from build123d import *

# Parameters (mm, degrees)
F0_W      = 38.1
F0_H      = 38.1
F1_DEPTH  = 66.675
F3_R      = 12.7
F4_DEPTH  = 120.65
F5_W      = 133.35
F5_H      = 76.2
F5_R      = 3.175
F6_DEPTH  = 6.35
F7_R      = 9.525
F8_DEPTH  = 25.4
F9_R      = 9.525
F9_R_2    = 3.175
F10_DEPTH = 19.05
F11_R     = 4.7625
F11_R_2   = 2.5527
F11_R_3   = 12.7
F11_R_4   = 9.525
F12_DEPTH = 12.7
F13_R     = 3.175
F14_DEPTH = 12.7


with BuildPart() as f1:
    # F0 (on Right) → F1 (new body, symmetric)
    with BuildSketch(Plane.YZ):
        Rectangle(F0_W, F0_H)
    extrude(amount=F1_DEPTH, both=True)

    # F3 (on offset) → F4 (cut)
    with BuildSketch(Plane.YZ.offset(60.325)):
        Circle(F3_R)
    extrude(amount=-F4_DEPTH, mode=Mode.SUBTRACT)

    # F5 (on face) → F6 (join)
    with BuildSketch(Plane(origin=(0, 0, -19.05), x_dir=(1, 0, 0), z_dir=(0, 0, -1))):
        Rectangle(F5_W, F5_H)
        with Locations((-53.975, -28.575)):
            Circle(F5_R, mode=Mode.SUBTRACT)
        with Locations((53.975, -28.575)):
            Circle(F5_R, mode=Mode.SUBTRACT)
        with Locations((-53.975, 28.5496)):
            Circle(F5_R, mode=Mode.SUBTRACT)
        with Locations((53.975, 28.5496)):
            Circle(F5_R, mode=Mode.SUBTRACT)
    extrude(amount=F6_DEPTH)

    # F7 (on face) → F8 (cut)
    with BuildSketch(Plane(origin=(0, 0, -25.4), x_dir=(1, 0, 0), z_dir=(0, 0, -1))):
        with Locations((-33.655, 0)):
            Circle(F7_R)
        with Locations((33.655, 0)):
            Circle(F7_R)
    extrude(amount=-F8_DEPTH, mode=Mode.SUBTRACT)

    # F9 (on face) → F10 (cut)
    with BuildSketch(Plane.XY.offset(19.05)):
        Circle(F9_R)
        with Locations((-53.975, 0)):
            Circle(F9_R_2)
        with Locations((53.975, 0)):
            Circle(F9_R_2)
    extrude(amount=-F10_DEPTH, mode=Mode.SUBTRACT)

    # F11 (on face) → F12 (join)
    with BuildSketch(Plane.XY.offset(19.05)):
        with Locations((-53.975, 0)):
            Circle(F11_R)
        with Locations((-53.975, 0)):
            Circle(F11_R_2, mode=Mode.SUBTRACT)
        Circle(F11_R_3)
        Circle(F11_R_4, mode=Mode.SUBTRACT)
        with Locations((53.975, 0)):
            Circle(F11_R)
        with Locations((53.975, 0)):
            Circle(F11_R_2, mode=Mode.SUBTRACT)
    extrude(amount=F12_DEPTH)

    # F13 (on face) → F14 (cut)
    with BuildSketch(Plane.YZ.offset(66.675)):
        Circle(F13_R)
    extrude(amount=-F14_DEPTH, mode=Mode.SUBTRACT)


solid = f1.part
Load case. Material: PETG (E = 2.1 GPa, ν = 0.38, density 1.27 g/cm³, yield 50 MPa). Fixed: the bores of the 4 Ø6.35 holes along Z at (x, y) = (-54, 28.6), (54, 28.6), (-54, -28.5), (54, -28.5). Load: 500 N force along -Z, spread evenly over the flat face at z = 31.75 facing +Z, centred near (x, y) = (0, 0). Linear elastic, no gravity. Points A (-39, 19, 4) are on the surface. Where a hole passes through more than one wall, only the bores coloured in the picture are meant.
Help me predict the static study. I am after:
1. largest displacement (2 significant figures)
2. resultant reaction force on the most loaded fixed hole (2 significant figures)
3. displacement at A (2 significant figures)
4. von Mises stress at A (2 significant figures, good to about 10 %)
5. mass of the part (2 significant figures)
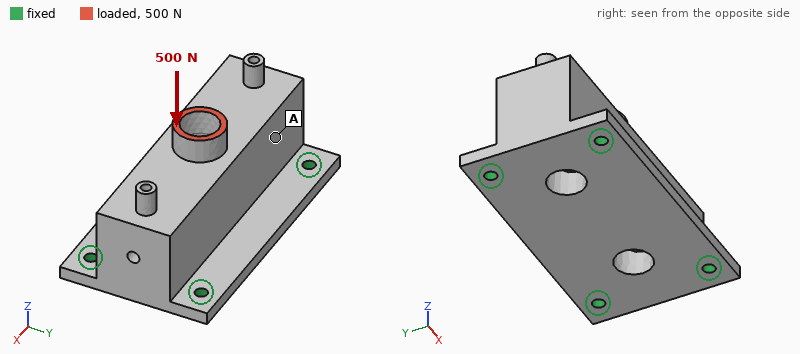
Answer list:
97 µm
150 N
42 µm
0.65 MPa
240 g
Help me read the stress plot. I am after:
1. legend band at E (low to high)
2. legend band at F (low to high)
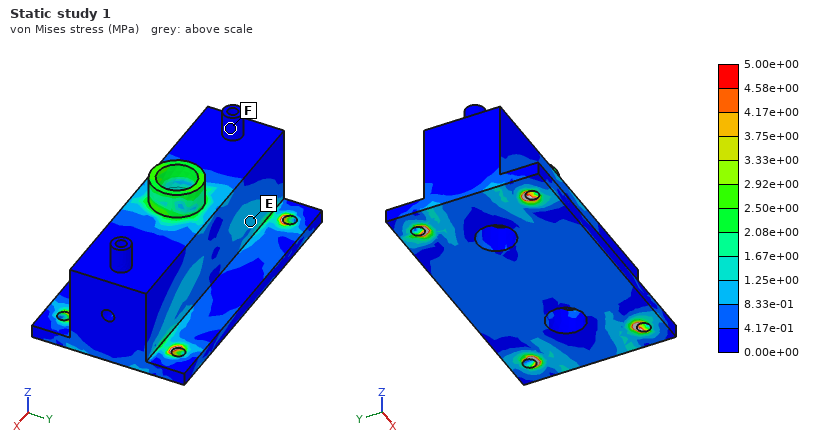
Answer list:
8.33e-01 to 1.25e+00 MPa
0.00e+00 to 4.17e-01 MPa
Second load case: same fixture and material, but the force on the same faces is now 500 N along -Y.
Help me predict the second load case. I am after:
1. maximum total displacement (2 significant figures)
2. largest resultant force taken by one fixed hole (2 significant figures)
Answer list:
0.44 mm
320 N
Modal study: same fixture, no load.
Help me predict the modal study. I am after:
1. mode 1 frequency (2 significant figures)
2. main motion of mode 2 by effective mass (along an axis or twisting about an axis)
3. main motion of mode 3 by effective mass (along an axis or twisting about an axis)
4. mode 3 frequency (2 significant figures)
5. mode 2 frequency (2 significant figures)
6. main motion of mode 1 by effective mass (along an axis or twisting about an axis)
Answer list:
1000 Hz
along Z
along X
1500 Hz
1200 Hz
along Y
